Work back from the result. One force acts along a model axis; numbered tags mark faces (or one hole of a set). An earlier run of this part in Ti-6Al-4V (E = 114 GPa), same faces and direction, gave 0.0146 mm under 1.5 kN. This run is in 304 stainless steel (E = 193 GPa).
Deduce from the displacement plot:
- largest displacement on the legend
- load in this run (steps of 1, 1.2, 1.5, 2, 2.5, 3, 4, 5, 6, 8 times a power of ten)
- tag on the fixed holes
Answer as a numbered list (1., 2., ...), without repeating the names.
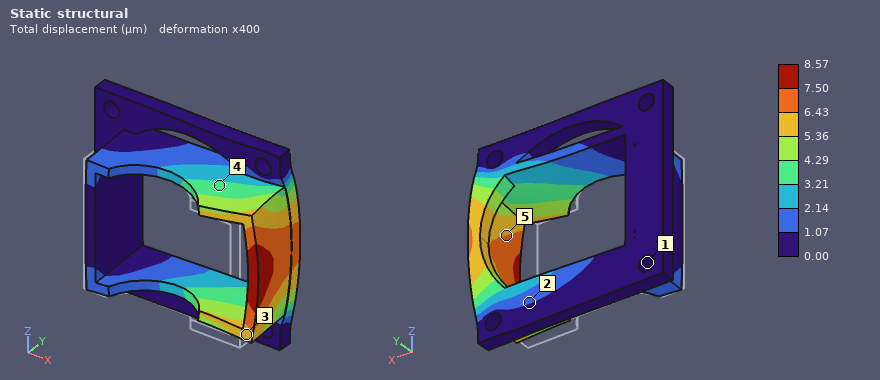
1. 8.57 µm
2. 1.5 kN
3. 1
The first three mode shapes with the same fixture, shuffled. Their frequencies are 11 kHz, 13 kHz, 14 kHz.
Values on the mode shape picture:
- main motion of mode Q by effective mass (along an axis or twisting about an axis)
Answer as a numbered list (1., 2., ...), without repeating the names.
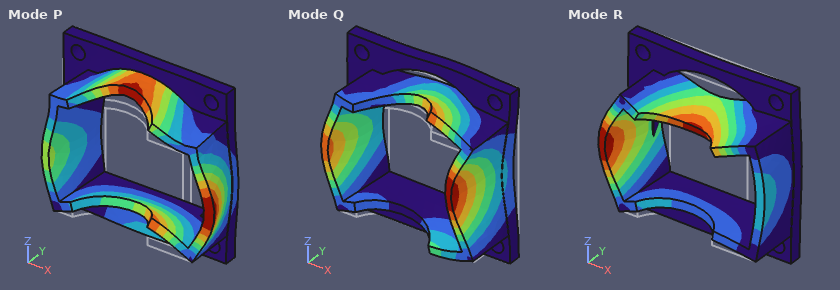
1. along X
